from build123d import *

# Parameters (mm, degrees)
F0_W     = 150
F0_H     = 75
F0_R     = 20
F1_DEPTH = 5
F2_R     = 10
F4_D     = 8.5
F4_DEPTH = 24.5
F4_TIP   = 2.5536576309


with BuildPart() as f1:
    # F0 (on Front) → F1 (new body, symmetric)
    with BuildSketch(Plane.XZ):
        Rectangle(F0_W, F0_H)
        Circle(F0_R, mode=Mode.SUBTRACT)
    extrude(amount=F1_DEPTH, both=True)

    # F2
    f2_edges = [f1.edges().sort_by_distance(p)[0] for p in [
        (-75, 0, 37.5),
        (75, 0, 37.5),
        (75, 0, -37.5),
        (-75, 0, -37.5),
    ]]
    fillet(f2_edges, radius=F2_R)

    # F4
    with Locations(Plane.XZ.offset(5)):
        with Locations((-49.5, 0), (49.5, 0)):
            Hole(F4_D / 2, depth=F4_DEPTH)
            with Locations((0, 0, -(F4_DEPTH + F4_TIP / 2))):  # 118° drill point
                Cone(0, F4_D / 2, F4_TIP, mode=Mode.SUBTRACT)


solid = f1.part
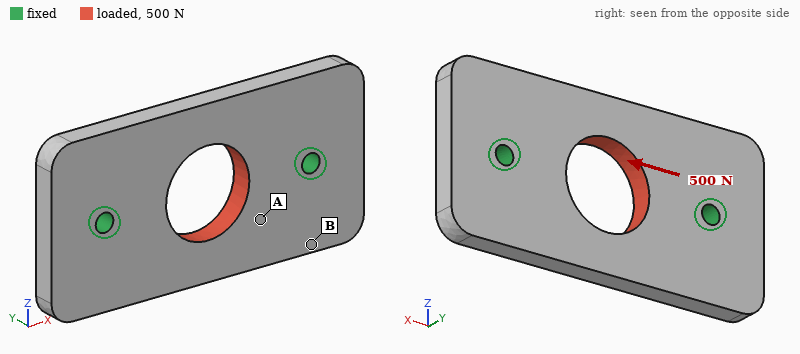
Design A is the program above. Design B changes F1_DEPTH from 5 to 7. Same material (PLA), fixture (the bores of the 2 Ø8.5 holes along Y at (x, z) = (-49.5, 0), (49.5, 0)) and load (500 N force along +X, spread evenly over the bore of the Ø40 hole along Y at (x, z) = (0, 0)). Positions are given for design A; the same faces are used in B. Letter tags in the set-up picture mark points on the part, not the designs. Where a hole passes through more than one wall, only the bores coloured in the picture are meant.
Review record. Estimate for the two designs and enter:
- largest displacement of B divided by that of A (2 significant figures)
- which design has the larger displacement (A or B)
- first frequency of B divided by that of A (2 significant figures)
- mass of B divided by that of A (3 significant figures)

0.71
A
1.3
1.40
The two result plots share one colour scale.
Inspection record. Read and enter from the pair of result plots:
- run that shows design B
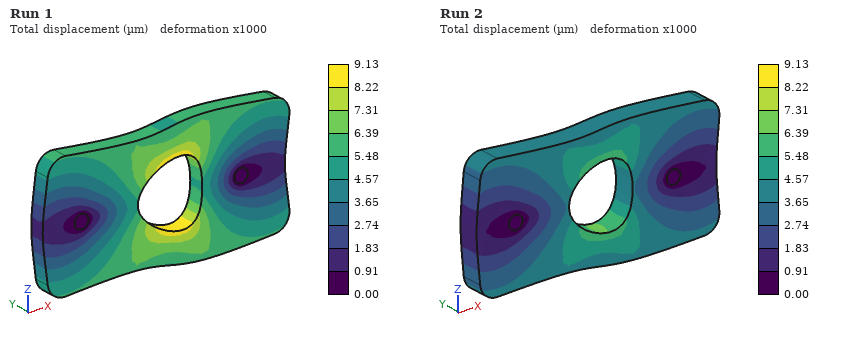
Run 2
